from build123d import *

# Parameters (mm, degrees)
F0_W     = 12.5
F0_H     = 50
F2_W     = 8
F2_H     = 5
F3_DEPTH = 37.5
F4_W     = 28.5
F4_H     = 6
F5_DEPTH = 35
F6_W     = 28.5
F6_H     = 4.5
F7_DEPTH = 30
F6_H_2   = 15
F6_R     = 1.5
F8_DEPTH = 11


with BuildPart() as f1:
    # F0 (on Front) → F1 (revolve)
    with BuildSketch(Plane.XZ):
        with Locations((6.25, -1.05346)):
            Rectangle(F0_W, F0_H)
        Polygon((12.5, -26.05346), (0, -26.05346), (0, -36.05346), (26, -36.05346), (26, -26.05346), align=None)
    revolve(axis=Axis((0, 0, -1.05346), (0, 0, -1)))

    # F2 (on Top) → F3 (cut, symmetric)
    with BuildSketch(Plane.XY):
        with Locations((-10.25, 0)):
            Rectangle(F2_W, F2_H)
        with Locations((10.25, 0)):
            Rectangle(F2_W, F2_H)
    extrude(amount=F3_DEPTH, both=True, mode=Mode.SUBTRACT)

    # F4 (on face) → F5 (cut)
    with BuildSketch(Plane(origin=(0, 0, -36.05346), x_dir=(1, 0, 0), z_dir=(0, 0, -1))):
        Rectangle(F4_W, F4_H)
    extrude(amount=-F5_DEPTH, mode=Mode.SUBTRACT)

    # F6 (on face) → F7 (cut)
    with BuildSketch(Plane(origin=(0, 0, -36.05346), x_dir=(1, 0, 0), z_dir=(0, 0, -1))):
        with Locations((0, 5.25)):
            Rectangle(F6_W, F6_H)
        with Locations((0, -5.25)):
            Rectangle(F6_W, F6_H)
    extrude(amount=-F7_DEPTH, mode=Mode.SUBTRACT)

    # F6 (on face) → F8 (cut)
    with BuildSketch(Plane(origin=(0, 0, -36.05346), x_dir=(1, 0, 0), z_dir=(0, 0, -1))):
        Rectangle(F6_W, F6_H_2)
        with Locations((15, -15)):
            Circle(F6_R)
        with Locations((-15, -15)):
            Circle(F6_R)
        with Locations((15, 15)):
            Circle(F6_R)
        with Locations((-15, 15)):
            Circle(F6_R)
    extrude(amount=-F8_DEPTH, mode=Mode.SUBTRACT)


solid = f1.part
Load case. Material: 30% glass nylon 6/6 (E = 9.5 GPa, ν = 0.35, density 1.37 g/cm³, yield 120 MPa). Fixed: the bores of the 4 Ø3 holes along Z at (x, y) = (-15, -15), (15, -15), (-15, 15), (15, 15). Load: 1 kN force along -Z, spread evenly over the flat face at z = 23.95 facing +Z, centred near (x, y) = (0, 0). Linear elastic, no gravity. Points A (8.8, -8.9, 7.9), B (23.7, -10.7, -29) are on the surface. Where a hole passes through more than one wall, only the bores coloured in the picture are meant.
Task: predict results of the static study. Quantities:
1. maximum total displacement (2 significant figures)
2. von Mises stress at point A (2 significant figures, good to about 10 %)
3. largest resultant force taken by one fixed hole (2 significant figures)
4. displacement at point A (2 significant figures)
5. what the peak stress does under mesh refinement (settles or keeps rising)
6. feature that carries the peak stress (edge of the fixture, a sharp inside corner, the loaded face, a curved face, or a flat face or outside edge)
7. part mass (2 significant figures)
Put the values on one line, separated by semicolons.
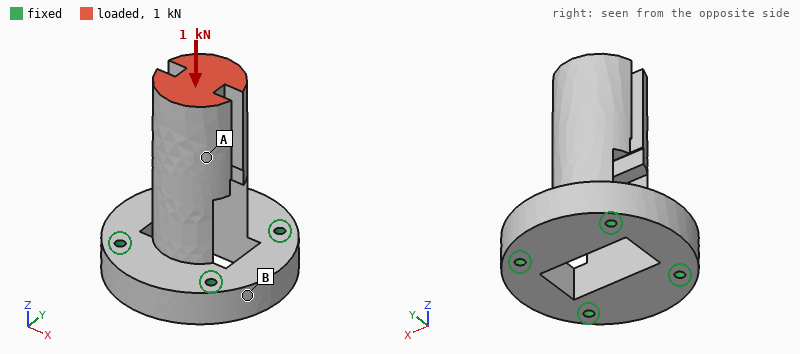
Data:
42 µm; 3.2 MPa; 250 N; 38 µm; keeps rising; edge of the fixture; 44 g
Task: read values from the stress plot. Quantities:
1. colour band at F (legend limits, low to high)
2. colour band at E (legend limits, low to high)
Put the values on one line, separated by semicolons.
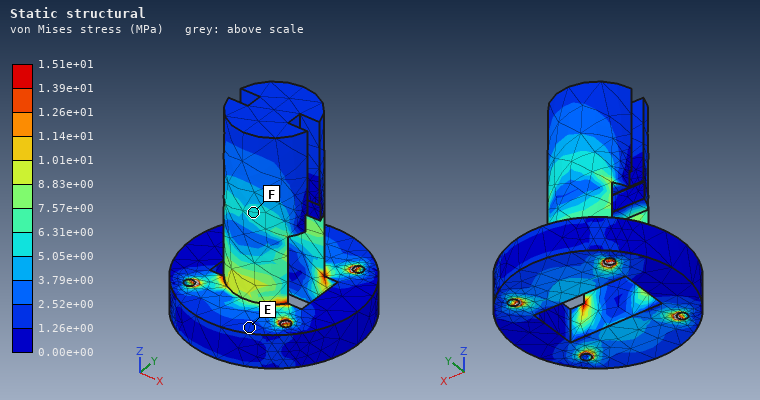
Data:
5.05e+00 to 6.31e+00 MPa; 1.26e+00 to 2.52e+00 MPa
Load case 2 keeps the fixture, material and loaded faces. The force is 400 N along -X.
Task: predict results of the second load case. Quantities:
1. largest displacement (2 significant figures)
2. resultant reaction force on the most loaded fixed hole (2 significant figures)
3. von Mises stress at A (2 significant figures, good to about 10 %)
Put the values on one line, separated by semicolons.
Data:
0.79 mm; 440 N; 5.4 MPa
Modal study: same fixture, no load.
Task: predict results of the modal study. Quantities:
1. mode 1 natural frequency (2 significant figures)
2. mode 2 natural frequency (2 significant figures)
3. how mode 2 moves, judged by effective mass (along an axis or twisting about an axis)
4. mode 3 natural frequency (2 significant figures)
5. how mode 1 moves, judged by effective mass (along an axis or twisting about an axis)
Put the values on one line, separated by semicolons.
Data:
1300 Hz; 1400 Hz; along Y; 3500 Hz; along X
